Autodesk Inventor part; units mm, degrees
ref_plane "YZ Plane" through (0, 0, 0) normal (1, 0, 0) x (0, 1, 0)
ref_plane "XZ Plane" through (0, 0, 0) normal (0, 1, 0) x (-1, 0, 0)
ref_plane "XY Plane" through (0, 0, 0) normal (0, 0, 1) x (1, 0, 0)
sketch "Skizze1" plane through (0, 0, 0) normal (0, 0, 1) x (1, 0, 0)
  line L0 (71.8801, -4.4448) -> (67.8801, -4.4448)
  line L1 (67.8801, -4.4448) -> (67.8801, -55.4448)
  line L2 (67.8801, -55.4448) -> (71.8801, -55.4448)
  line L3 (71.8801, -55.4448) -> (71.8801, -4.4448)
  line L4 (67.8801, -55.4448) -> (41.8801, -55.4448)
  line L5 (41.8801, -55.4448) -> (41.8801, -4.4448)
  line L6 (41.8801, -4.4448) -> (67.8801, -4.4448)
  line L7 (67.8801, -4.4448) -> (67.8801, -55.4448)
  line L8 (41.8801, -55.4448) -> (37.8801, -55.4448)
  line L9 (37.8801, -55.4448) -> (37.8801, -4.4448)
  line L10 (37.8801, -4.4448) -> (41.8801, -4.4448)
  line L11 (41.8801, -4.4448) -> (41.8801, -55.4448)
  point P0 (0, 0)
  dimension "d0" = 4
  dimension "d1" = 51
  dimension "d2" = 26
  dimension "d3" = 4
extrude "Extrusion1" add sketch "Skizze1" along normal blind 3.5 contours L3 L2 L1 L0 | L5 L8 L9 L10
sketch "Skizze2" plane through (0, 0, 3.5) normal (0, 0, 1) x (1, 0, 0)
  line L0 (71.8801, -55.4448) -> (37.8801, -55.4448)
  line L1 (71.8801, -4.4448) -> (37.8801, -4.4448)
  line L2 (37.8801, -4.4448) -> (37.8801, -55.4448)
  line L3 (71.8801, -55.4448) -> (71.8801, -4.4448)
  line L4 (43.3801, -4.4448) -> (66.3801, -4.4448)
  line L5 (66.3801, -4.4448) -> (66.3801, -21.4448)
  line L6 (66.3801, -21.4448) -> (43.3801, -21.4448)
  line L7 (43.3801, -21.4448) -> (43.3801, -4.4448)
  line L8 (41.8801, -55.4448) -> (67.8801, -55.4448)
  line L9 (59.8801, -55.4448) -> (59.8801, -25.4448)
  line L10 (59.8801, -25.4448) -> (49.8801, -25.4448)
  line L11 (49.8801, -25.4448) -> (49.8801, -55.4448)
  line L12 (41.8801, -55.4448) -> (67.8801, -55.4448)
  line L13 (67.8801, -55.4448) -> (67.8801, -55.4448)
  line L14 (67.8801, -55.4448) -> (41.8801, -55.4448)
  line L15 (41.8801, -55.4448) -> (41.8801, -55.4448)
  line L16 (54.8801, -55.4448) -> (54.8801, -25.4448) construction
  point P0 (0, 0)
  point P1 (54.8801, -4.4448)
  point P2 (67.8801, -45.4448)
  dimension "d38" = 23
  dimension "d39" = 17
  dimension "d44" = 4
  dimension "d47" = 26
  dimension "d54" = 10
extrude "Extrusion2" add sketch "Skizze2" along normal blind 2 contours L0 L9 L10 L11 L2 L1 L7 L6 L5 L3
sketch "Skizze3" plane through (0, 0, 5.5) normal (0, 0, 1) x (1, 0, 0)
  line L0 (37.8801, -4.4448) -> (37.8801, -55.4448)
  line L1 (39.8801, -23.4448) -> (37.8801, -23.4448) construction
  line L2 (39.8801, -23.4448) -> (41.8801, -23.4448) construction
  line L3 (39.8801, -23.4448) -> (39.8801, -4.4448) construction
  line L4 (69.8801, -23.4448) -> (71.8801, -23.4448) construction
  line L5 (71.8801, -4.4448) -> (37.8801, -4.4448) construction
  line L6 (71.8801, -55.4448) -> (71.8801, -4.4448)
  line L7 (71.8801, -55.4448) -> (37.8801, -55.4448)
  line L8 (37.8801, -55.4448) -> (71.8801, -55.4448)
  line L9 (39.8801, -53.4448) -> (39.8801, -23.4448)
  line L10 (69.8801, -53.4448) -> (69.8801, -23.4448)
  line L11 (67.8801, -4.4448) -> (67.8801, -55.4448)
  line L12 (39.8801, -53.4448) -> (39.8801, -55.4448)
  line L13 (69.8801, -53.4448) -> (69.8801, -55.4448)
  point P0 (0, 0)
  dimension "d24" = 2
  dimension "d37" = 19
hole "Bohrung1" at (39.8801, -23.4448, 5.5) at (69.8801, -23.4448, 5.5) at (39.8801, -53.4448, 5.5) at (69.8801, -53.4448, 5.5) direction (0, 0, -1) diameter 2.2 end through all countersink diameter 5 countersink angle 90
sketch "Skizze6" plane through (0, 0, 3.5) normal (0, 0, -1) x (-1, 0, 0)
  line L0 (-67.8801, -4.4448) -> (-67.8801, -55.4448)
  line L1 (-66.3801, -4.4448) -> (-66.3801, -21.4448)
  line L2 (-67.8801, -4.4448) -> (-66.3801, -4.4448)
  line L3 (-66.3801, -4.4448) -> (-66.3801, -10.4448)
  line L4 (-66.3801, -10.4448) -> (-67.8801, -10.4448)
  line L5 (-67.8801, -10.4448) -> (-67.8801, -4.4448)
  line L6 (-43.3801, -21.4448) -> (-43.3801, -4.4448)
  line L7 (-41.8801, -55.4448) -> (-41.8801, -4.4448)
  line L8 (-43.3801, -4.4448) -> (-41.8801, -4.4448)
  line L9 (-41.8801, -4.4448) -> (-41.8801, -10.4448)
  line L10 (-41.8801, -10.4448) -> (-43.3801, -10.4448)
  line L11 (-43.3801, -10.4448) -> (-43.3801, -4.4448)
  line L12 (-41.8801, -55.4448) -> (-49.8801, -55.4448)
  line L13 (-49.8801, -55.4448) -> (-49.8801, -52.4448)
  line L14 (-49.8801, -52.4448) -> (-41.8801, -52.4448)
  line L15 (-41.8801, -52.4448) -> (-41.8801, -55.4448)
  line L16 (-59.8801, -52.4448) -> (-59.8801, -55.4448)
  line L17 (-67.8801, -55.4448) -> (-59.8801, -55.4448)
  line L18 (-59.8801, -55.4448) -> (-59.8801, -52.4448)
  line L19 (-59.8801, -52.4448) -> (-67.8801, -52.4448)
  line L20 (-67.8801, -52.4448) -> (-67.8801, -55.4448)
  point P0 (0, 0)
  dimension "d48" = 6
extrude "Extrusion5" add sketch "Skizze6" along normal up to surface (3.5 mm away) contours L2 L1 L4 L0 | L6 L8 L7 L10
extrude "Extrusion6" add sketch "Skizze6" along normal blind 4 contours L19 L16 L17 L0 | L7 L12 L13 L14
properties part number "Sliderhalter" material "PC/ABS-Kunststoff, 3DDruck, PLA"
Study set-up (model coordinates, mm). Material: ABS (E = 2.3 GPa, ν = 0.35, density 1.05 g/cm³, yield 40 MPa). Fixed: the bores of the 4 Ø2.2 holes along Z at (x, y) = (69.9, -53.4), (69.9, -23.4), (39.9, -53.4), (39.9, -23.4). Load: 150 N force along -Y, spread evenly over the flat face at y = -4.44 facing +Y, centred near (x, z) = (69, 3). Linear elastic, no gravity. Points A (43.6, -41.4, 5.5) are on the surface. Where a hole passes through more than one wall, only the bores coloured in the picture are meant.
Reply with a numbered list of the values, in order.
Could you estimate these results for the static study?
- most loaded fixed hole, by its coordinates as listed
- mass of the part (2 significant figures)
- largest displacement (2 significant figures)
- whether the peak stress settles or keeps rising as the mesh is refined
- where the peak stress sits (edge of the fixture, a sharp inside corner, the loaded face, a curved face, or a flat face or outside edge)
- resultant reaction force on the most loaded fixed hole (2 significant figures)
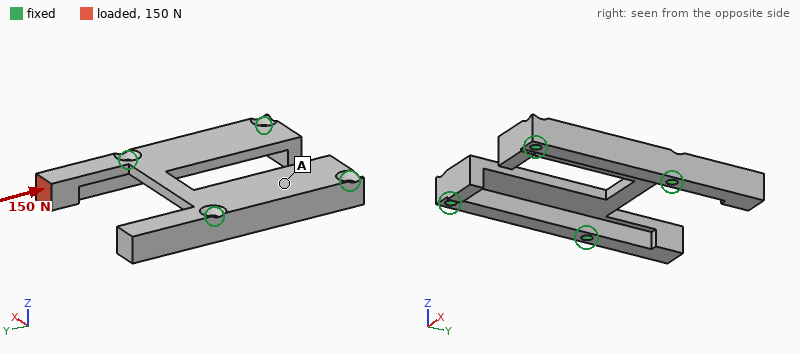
1. (69.9, -23.4)
2. 3.8 g
3. 0.15 mm
4. keeps rising
5. edge of the fixture
6. 140 N
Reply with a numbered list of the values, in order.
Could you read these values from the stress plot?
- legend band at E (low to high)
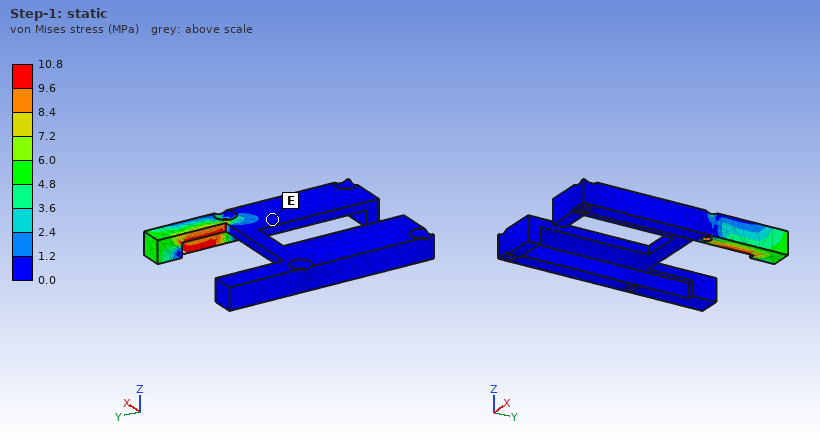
1. 0.0 to 1.2 MPa
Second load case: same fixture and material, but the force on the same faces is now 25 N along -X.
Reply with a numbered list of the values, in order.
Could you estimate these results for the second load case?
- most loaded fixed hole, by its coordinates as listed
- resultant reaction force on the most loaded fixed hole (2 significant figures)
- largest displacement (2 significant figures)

1. (69.9, -23.4)
2. 32 N
3. 0.63 mm
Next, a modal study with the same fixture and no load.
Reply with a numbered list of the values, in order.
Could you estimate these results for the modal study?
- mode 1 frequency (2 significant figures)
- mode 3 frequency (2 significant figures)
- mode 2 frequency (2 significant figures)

1. 2500 Hz
2. 3200 Hz
3. 2500 Hz
